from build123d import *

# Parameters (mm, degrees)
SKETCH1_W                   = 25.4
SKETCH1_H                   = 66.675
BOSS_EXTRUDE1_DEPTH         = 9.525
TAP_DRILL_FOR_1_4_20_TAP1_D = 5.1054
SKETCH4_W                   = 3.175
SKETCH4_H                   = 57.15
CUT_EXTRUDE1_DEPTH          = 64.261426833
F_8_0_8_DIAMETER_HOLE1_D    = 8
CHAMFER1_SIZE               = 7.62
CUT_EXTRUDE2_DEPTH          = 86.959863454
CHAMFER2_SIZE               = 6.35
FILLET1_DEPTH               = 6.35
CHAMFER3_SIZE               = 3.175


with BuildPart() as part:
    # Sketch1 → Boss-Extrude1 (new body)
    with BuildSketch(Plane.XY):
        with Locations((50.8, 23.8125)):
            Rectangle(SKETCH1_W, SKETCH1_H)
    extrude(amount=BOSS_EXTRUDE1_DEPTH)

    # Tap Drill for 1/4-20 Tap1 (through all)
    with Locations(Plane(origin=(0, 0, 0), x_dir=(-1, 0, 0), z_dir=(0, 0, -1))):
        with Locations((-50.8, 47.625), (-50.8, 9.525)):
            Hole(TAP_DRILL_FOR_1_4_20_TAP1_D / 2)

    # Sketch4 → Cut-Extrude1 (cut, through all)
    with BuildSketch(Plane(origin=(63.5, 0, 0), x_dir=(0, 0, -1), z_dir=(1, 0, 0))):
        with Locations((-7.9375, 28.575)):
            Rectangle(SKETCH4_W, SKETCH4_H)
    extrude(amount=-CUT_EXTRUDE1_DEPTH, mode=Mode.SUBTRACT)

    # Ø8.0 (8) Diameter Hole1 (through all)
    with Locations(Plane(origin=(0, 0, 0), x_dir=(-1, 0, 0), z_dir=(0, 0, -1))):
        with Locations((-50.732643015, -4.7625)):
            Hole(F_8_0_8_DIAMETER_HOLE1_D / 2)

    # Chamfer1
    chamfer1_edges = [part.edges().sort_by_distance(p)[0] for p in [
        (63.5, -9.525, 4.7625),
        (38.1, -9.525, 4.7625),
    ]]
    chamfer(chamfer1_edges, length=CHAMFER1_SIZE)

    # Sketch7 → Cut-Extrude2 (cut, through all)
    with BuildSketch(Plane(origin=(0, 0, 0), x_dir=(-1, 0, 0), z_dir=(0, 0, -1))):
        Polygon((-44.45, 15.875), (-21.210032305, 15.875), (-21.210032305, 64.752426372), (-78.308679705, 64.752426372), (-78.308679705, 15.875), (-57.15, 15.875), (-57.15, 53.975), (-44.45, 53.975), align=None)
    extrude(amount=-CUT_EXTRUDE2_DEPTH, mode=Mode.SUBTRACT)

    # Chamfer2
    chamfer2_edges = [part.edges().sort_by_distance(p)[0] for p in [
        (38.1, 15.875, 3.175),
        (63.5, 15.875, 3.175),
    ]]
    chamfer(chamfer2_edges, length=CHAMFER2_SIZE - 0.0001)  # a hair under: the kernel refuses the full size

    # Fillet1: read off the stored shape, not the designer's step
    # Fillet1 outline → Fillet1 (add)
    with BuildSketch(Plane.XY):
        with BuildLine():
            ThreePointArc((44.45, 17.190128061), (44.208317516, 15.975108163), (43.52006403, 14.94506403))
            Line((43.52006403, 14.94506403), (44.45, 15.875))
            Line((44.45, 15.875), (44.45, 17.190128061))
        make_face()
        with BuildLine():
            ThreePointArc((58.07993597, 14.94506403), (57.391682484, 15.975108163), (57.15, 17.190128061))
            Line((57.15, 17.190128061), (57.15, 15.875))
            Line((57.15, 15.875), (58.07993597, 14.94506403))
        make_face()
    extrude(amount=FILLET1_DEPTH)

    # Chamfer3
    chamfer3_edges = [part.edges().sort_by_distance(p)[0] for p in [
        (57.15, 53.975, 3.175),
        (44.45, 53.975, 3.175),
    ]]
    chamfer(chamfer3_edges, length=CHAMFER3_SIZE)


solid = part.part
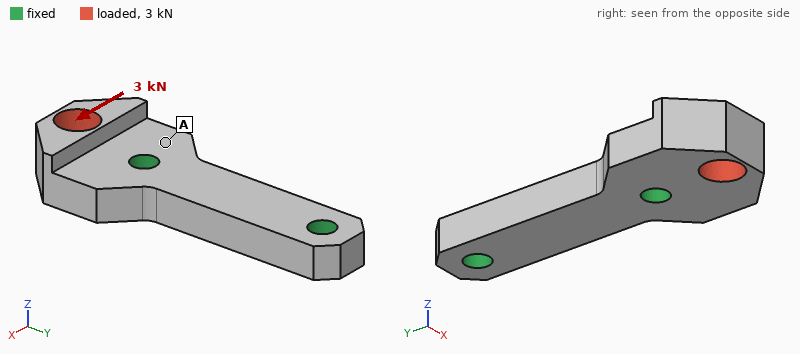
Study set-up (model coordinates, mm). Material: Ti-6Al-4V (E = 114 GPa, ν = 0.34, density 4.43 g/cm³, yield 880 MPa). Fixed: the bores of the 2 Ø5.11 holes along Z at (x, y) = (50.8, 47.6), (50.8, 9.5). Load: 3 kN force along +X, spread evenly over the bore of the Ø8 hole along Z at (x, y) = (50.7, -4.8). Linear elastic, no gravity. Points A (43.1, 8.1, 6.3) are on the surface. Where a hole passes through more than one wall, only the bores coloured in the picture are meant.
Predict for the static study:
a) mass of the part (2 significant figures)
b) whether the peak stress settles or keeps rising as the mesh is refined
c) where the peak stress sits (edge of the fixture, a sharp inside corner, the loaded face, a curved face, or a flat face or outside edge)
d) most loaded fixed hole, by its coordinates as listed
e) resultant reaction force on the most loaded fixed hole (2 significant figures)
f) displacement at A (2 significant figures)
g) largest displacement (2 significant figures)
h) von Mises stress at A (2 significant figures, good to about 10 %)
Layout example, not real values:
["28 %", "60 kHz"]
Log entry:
["28 g", "keeps rising", "edge of the fixture", "(50.8, 9.5)", "3.5 kN", "9.7 µm", "46 µm", "47 MPa"]
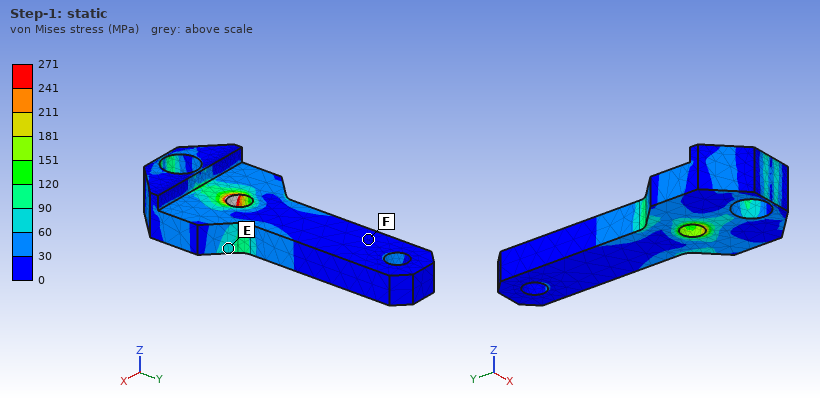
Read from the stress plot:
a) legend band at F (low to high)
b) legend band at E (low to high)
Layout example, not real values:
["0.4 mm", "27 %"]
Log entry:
["0 to 30 MPa", "60 to 90 MPa"]
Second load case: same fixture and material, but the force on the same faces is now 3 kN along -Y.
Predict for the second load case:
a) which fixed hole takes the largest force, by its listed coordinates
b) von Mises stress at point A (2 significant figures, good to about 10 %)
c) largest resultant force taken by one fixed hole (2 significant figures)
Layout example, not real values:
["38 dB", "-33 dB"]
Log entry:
["(50.8, 9.5)", "32 MPa", "2.8 kN"]
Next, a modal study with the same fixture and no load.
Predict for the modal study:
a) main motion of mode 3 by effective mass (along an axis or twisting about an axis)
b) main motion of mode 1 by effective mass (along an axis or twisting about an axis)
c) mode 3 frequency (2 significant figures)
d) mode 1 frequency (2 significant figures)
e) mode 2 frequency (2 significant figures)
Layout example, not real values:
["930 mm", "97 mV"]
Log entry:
["twisting about Y", "along Z", "19 kHz", "14 kHz", "17 kHz"]
